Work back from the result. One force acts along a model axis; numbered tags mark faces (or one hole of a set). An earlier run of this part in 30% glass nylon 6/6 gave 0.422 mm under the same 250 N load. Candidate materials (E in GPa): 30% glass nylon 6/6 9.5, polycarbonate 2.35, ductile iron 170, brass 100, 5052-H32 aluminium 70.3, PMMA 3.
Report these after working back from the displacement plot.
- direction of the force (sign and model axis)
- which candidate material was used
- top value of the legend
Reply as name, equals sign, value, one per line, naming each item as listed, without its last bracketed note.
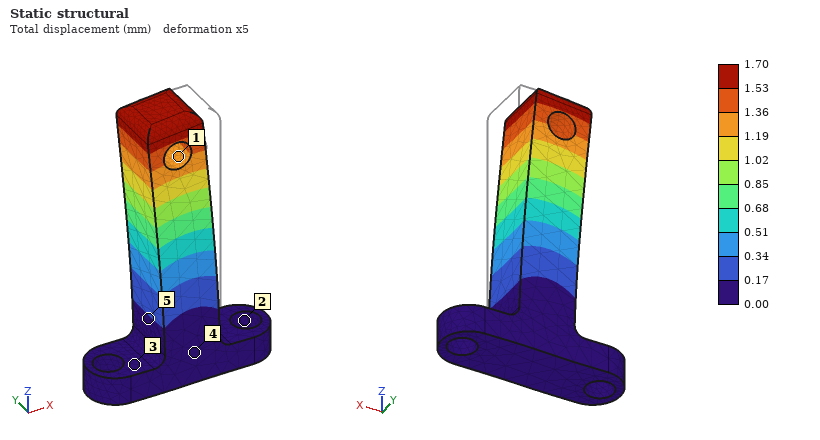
direction of the force = -X
which candidate material was used = polycarbonate
top value of the legend = 1.70 mm
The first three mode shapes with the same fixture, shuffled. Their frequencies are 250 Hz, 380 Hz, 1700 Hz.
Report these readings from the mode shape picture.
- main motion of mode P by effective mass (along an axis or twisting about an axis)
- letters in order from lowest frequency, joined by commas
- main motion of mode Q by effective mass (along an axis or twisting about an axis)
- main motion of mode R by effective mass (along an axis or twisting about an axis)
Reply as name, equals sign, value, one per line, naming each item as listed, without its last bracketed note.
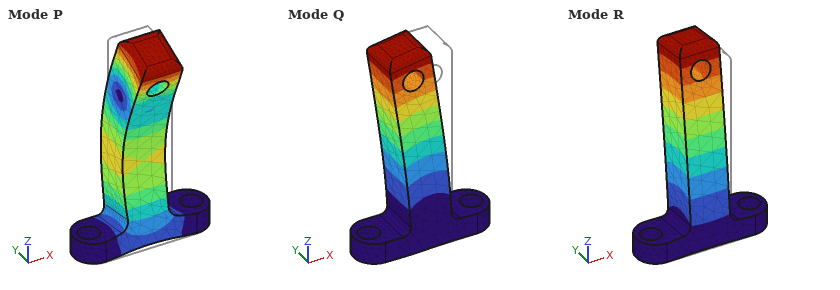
main motion of mode P by effective mass = along Y
letters in order from lowest frequency, joined by commas = R, Q, P
main motion of mode Q by effective mass = along X
main motion of mode R by effective mass = along Y
